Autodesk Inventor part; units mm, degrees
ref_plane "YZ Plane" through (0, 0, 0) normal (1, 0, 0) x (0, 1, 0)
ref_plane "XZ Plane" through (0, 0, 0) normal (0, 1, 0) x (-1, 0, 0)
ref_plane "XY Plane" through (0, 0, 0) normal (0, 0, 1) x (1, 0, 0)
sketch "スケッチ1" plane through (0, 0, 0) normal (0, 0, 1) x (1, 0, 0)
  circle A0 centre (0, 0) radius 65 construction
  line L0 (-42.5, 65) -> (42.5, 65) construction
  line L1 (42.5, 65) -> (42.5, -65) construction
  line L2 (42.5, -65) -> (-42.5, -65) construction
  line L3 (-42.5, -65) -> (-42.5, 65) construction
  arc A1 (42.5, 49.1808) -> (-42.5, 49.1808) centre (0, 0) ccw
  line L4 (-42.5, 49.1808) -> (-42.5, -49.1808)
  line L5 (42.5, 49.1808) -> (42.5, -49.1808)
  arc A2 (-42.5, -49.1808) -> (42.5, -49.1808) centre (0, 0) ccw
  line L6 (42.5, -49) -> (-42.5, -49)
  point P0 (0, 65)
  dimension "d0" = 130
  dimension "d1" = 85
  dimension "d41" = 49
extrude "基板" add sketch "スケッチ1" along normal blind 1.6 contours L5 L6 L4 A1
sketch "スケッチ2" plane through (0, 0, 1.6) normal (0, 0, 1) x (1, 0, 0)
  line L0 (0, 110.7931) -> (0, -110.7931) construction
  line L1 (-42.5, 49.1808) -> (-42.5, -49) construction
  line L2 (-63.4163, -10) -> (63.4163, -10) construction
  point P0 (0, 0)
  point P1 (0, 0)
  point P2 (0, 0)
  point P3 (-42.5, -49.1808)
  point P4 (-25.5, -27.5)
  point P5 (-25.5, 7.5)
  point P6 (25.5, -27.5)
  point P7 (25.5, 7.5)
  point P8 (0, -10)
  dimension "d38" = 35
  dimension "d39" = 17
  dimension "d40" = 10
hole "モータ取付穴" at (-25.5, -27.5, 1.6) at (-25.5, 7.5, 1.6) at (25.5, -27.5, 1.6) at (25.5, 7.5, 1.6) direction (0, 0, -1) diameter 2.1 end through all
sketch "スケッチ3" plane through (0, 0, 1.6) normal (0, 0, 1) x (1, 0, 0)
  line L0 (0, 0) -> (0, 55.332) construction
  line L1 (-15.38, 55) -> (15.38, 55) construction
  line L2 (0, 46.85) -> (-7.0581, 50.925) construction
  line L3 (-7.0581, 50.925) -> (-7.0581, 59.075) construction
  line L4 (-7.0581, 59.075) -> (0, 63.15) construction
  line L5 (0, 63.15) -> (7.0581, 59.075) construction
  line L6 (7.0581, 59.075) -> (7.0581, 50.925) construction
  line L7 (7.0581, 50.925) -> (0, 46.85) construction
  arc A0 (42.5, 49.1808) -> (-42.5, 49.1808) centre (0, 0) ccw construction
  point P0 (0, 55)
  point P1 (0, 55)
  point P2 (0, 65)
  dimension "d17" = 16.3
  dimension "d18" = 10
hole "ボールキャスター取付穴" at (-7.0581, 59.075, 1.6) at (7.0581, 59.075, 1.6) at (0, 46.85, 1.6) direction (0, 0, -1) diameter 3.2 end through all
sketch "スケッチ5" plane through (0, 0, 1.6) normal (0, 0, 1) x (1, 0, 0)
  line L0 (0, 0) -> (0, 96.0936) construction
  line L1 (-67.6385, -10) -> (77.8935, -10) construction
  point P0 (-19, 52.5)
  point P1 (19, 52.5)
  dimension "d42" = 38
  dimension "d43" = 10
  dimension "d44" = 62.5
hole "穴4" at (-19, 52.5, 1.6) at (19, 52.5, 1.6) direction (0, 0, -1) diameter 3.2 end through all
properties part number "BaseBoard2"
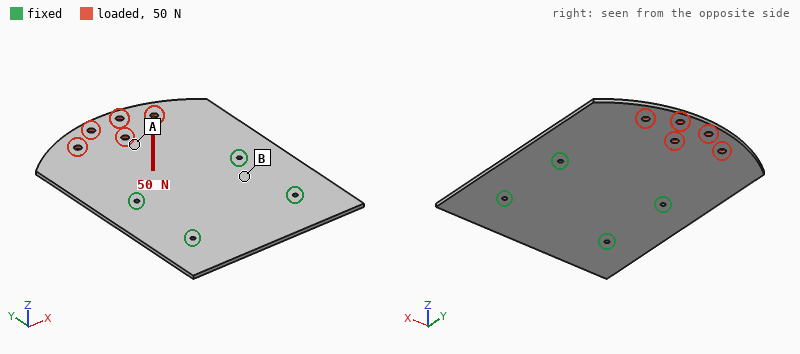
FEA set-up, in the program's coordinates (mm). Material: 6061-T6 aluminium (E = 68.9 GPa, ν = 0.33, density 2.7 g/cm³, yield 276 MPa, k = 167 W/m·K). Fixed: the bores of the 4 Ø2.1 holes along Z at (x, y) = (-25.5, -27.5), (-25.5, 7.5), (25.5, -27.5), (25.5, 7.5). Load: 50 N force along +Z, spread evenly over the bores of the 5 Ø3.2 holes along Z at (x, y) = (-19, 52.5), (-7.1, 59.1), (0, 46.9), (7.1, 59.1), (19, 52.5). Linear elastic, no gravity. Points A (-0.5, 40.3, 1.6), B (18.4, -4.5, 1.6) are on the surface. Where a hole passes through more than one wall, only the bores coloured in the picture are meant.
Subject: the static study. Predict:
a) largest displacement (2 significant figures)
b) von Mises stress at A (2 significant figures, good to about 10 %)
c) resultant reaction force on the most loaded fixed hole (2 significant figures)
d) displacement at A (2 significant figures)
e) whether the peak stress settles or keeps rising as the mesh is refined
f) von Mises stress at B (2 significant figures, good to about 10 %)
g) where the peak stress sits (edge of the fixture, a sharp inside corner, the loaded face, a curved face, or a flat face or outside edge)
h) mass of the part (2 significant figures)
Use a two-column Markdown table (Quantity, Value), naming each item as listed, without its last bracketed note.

| Quantity | Value |
|---|---|
| largest displacement | 1.4 mm |
| von Mises stress at A | 25 MPa |
| resultant reaction force on the most loaded fixed hole | 40 N |
| displacement at A | 0.66 mm |
| whether the peak stress settles or keeps rising as the mesh is refined | keeps rising |
| von Mises stress at B | 11 MPa |
| where the peak stress sits | edge of the fixture |
| mass of the part | 40 g |
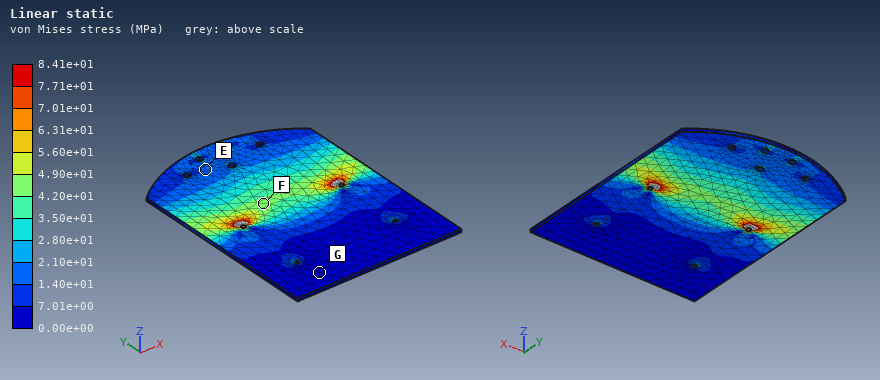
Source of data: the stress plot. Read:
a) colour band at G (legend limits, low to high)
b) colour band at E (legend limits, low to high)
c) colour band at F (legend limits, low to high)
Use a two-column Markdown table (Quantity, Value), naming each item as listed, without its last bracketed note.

| Quantity | Value |
|---|---|
| colour band at G | 0.00e+00 to 7.01e+00 MPa |
| colour band at E | 1.40e+01 to 2.10e+01 MPa |
| colour band at F | 4.20e+01 to 4.90e+01 MPa |
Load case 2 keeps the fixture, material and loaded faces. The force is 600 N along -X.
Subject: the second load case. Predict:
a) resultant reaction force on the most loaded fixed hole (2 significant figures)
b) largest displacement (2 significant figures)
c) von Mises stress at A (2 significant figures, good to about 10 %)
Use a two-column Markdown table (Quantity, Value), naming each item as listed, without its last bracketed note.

| Quantity | Value |
|---|---|
| resultant reaction force on the most loaded fixed hole | 480 N |
| largest displacement | 21 µm |
| von Mises stress at A | 13 MPa |
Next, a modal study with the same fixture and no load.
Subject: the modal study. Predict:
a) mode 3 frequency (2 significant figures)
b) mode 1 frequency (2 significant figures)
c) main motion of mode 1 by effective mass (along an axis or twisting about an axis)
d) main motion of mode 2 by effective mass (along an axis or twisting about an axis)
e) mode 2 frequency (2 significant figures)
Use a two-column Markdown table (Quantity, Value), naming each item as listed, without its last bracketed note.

| Quantity | Value |
|---|---|
| mode 3 frequency | 1700 Hz |
| mode 1 frequency | 420 Hz |
| main motion of mode 1 by effective mass | along Z |
| main motion of mode 2 by effective mass | twisting about Y |
| mode 2 frequency | 880 Hz |
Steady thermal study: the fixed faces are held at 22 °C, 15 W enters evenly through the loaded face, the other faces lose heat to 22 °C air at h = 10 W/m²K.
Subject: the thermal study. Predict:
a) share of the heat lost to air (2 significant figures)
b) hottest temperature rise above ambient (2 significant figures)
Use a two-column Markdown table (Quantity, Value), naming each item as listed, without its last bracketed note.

| Quantity | Value |
|---|---|
| share of the heat lost to air | 15 % |
| hottest temperature rise above ambient | 42 K |
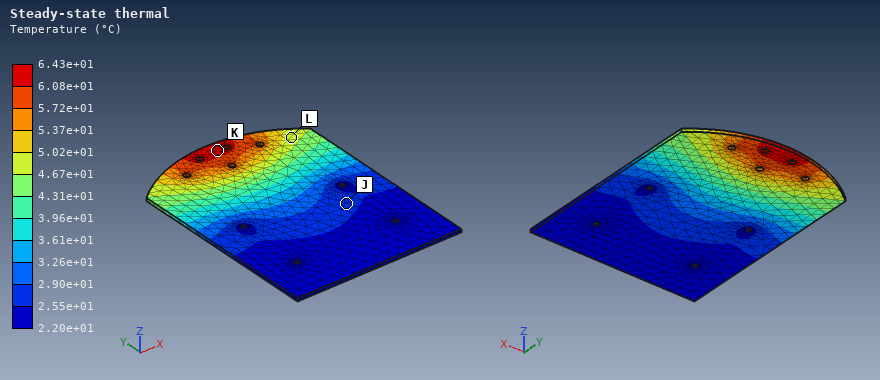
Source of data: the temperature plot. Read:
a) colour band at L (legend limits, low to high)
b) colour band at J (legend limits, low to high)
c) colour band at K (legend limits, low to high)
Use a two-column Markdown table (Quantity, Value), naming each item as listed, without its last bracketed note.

| Quantity | Value |
|---|---|
| colour band at L | 4.67e+01 to 5.02e+01 °C |
| colour band at J | 2.55e+01 to 2.90e+01 °C |
| colour band at K | 6.08e+01 to 6.43e+01 °C |
